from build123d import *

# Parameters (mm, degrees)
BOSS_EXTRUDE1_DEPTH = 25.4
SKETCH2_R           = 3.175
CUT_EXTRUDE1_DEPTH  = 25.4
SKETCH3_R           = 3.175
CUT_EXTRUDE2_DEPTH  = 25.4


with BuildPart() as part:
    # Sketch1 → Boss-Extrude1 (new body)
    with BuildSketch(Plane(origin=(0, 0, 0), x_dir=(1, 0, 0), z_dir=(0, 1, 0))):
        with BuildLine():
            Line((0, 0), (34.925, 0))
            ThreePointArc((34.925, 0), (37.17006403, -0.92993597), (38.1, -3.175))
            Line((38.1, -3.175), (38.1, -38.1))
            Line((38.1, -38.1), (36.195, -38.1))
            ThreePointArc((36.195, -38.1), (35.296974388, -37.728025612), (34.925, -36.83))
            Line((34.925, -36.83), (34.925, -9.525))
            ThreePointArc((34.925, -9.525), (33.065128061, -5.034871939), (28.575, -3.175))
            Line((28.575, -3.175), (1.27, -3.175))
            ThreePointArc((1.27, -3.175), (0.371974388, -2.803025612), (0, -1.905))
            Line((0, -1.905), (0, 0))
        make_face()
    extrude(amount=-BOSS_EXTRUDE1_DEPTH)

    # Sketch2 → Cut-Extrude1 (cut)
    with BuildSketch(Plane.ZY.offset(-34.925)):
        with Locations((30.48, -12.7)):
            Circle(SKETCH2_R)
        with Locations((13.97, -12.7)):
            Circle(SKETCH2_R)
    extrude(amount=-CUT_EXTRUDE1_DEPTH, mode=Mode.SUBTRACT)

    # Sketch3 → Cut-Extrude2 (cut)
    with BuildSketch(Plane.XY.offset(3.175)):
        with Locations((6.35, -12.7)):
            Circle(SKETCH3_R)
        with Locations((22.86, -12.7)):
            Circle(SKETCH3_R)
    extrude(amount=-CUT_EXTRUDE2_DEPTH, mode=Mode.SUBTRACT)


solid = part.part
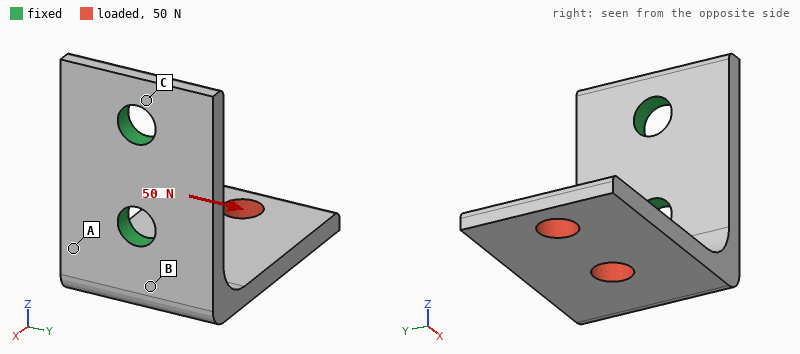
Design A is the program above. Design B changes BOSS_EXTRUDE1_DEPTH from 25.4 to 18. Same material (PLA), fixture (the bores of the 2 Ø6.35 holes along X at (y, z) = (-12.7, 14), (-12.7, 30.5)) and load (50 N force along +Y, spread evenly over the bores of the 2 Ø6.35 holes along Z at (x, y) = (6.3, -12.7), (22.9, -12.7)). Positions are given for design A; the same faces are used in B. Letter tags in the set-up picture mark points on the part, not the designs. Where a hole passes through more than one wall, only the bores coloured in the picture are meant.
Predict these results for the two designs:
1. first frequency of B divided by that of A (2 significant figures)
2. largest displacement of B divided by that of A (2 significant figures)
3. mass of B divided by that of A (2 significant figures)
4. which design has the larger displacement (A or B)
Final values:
1.0
1.5
0.69
B
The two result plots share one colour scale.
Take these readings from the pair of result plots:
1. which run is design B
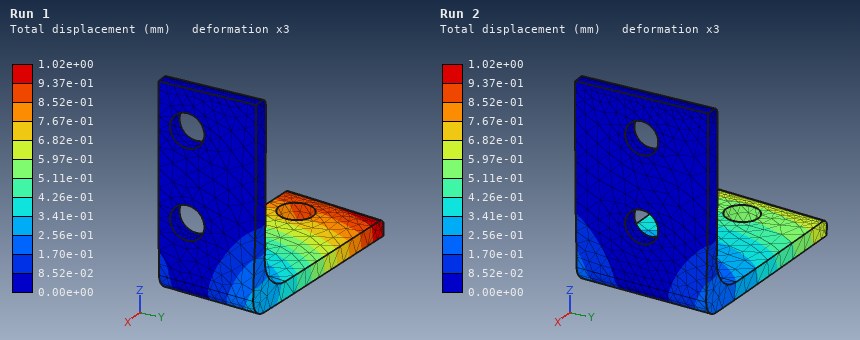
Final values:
Run 1
